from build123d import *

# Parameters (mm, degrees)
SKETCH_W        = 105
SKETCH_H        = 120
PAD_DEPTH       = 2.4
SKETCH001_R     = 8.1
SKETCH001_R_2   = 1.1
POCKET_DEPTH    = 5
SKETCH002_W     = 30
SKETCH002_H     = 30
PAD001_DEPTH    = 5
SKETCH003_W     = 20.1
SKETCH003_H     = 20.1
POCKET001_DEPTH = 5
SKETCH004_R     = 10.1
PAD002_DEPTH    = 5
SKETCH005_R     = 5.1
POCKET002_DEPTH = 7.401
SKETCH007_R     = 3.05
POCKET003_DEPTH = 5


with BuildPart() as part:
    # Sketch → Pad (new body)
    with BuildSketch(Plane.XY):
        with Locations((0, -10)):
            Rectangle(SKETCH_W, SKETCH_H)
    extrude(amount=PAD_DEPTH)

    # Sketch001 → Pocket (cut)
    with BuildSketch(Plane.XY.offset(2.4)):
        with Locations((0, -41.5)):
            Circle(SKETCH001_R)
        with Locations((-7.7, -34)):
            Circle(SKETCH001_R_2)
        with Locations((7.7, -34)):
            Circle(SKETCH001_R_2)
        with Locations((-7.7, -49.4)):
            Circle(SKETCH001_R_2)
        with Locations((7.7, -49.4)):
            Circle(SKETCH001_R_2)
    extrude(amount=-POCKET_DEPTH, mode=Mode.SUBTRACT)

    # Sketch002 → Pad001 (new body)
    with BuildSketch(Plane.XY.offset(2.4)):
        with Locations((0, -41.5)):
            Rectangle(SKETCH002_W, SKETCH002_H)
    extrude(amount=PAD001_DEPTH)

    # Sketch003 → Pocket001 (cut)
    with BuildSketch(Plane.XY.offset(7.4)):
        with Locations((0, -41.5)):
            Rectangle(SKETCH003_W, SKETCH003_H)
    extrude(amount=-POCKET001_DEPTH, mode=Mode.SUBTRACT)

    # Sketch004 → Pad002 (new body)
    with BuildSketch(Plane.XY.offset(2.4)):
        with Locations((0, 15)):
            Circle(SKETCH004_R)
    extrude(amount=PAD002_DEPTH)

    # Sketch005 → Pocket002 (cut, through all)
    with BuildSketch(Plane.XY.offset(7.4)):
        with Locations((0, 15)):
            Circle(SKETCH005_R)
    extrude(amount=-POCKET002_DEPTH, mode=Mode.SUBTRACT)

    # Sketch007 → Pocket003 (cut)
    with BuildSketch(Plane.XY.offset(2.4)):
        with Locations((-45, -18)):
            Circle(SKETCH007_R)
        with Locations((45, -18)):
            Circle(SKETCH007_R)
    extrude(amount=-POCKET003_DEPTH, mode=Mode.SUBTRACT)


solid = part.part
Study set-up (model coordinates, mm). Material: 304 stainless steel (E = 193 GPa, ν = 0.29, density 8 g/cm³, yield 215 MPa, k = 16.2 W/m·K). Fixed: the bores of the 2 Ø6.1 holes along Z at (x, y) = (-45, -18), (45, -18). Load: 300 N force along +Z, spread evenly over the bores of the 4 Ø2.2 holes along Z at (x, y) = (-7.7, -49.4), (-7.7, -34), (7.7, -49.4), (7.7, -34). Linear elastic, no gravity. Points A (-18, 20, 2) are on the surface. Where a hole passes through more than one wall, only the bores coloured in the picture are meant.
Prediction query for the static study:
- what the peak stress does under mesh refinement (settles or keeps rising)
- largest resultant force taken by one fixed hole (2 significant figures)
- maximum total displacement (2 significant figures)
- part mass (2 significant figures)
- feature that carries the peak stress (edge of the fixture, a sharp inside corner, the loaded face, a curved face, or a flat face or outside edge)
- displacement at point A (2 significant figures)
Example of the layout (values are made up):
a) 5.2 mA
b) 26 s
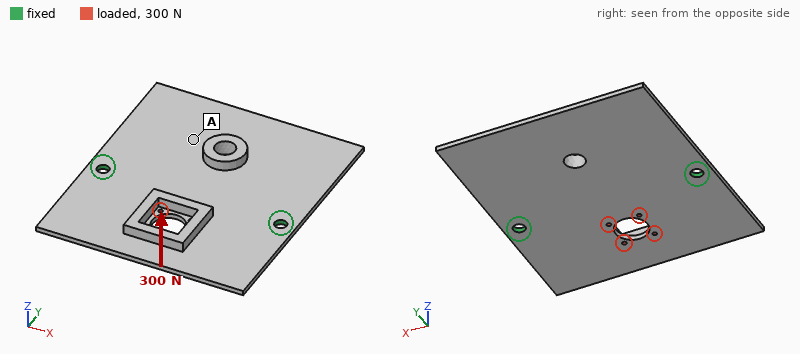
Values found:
a) keeps rising
b) 200 N
c) 0.32 mm
d) 260 g
e) edge of the fixture
f) 0.075 mm
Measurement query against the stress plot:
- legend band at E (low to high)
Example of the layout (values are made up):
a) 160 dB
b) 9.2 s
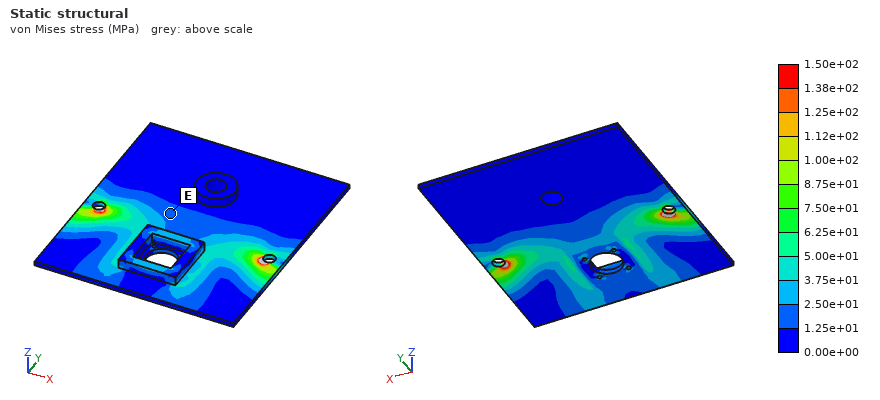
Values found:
a) 1.25e+01 to 2.50e+01 MPa
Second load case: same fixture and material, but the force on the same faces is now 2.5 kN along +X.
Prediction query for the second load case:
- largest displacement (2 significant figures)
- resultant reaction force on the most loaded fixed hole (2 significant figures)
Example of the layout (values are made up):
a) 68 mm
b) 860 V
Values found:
a) 8.9 µm
b) 1.4 kN
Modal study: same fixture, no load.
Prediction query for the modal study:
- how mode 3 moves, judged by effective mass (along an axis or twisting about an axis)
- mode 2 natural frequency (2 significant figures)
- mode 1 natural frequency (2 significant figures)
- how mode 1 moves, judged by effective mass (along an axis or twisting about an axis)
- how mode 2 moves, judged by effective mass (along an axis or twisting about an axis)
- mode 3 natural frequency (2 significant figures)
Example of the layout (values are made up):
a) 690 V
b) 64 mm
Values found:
a) twisting about Y
b) 630 Hz
c) 340 Hz
d) along Z
e) along Z
f) 820 Hz
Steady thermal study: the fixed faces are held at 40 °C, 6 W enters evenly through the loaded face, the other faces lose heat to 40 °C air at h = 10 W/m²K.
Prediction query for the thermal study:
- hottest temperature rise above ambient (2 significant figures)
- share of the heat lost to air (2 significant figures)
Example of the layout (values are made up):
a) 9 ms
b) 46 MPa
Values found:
a) 52 K
b) 65 %
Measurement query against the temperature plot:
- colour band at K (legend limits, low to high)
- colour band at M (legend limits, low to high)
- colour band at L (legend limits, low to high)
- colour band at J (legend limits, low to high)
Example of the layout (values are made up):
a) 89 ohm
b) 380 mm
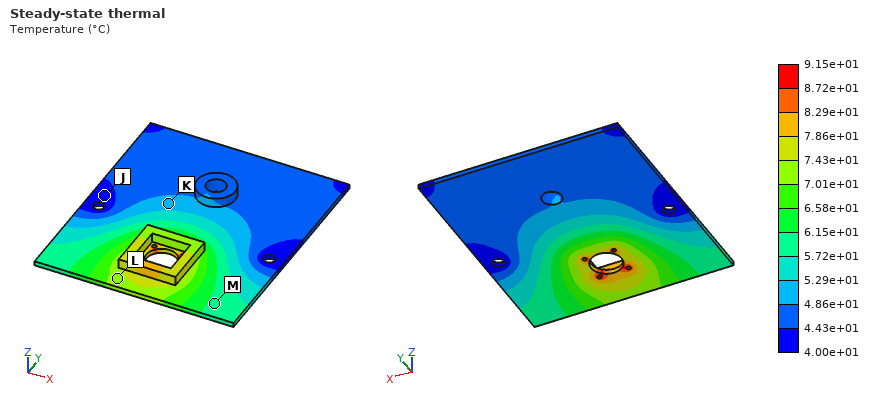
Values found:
a) 4.86e+01 to 5.29e+01 °C
b) 5.72e+01 to 6.15e+01 °C
c) 7.01e+01 to 7.43e+01 °C
d) 4.00e+01 to 4.43e+01 °C
